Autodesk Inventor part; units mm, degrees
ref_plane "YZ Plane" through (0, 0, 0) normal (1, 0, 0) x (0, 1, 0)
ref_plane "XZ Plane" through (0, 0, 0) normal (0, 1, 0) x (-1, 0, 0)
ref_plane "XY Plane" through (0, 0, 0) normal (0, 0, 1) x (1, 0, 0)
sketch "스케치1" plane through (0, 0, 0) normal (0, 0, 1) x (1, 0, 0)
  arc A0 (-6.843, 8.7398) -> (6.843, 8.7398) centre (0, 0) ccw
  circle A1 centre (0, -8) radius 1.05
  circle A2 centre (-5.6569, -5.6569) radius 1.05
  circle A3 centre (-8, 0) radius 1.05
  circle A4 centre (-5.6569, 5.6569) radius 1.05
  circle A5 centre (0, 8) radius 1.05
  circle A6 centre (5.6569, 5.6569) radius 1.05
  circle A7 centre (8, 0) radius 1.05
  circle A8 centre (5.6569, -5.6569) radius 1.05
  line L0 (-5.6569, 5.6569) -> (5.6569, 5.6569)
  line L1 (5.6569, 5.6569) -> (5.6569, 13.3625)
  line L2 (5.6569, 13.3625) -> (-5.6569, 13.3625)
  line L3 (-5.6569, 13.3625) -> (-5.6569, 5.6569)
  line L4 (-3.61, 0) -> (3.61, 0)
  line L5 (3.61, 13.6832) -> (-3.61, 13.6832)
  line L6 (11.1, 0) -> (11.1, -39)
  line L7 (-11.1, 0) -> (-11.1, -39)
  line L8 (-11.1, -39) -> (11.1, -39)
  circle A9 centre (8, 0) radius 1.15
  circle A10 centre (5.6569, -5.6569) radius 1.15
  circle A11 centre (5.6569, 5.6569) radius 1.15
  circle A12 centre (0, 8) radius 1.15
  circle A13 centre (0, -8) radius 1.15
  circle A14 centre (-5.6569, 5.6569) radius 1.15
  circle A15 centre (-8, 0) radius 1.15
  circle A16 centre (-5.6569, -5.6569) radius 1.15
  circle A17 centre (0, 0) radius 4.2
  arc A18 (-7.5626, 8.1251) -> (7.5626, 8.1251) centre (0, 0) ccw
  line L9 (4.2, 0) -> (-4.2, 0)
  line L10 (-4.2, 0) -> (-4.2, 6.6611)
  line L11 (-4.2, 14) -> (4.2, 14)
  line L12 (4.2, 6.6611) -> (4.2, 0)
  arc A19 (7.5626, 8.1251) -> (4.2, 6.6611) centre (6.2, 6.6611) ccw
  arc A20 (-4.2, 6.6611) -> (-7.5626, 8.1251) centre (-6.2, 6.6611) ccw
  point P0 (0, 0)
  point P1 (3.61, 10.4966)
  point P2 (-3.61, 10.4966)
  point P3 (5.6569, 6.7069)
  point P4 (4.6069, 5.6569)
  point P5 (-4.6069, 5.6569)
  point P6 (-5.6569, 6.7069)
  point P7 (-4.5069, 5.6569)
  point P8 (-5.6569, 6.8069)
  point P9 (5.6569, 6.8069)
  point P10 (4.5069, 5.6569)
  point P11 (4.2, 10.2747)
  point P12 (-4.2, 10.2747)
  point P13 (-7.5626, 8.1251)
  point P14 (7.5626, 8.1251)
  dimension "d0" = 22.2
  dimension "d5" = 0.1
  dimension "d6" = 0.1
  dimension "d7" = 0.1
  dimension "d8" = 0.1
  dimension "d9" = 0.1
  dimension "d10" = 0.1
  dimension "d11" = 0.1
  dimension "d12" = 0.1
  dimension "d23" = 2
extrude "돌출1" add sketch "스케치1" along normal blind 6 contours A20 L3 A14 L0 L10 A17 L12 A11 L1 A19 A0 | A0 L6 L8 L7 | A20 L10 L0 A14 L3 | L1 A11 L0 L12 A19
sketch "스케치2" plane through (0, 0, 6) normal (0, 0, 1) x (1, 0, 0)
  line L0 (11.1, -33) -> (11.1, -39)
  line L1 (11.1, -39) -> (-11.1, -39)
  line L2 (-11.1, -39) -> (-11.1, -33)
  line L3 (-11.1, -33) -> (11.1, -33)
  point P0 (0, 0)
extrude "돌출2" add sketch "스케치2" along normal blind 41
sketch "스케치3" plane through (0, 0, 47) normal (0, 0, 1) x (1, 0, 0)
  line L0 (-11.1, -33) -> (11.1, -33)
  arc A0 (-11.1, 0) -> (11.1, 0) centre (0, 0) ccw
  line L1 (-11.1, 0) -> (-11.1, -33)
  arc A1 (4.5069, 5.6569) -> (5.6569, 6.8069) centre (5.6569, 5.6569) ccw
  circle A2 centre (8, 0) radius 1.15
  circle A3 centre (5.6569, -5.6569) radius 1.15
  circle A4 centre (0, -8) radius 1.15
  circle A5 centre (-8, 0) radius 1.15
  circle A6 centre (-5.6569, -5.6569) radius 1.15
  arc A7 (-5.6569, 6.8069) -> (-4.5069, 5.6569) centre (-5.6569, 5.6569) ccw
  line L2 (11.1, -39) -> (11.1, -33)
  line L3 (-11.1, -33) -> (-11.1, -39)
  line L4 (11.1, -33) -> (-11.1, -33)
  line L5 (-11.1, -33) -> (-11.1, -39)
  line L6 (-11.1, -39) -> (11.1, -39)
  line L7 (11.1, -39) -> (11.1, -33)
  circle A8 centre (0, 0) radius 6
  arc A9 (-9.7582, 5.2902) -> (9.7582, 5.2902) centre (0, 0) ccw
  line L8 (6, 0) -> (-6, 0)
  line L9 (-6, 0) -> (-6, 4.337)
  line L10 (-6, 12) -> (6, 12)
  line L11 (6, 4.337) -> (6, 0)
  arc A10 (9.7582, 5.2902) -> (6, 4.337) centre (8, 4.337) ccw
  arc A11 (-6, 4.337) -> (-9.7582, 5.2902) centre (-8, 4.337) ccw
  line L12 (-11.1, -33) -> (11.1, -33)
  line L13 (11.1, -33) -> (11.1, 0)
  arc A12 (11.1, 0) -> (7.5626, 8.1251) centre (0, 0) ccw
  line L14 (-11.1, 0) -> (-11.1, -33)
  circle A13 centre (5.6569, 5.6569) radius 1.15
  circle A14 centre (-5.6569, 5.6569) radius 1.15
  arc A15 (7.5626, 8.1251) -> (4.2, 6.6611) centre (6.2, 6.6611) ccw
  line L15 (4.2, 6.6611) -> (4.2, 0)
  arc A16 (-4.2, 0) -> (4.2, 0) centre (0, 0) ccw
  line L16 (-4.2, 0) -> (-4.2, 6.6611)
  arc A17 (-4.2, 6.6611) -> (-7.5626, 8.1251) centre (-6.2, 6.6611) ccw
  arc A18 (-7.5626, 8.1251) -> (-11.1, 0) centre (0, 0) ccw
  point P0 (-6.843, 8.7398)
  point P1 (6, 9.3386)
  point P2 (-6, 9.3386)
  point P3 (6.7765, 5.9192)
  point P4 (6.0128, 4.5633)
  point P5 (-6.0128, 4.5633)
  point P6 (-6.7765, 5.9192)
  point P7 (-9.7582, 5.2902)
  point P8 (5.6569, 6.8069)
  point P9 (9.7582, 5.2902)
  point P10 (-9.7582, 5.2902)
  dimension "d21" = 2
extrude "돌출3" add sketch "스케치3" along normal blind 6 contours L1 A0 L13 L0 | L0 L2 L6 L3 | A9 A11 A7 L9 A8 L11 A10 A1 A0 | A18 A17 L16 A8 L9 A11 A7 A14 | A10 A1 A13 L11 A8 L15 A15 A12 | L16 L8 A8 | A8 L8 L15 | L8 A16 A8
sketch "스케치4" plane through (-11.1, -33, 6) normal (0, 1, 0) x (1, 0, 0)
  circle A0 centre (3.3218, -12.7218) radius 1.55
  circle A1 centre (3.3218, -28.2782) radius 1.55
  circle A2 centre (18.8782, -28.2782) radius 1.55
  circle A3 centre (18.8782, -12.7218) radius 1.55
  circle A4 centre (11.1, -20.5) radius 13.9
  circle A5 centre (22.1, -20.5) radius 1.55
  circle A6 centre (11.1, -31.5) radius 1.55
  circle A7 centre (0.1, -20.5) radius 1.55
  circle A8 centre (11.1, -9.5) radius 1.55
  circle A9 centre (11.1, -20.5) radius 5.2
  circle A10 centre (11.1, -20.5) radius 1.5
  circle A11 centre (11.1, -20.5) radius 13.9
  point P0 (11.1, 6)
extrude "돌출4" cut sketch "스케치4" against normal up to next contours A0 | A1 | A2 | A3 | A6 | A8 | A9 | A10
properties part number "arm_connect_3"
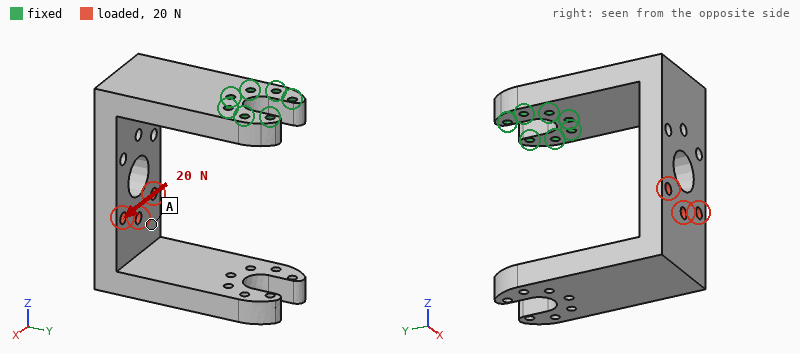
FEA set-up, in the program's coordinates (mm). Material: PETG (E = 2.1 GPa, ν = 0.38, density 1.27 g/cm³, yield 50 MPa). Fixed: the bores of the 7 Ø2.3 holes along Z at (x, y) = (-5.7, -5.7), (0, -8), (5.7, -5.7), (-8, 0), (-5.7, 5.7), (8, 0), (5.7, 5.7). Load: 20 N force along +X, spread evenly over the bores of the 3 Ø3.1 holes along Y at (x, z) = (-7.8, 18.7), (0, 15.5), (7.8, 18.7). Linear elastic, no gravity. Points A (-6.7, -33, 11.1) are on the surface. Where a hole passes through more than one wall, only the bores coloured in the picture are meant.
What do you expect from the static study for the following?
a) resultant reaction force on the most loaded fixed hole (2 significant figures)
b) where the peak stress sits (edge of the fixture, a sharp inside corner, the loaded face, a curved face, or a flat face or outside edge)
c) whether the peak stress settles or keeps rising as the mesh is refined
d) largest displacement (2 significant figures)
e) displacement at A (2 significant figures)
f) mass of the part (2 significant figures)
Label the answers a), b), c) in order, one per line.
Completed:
a) 40 N
b) edge of the fixture
c) keeps rising
d) 0.84 mm
e) 0.63 mm
f) 20 g
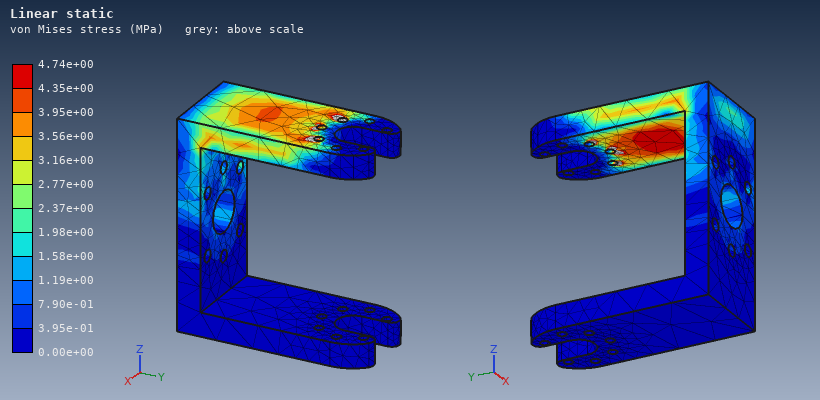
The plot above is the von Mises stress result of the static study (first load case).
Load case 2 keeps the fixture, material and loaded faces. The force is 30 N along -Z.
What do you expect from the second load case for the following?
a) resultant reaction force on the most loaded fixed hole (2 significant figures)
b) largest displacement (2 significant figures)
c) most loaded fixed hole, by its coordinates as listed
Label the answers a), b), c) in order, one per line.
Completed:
a) 48 N
b) 0.81 mm
c) (0, -8)
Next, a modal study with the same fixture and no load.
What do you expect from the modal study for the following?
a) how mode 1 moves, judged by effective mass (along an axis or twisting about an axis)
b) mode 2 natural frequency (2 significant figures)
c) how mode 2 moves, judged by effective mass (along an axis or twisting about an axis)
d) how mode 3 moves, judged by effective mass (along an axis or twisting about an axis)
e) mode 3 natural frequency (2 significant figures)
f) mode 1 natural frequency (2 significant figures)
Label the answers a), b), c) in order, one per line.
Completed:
a) along Y
b) 200 Hz
c) along X
d) along Z
e) 380 Hz
f) 140 Hz
